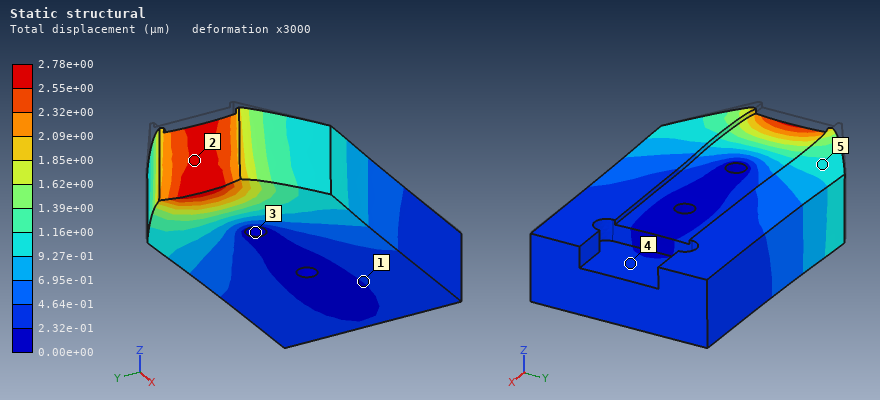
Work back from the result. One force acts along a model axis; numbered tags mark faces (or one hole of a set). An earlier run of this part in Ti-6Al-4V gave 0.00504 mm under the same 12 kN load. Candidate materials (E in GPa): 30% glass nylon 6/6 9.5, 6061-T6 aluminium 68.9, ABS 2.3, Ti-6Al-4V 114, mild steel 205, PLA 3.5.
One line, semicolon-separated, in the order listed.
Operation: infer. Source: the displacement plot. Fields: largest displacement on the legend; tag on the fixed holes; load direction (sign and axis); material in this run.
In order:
2.78e+00 µm; 3; +X; mild steel
